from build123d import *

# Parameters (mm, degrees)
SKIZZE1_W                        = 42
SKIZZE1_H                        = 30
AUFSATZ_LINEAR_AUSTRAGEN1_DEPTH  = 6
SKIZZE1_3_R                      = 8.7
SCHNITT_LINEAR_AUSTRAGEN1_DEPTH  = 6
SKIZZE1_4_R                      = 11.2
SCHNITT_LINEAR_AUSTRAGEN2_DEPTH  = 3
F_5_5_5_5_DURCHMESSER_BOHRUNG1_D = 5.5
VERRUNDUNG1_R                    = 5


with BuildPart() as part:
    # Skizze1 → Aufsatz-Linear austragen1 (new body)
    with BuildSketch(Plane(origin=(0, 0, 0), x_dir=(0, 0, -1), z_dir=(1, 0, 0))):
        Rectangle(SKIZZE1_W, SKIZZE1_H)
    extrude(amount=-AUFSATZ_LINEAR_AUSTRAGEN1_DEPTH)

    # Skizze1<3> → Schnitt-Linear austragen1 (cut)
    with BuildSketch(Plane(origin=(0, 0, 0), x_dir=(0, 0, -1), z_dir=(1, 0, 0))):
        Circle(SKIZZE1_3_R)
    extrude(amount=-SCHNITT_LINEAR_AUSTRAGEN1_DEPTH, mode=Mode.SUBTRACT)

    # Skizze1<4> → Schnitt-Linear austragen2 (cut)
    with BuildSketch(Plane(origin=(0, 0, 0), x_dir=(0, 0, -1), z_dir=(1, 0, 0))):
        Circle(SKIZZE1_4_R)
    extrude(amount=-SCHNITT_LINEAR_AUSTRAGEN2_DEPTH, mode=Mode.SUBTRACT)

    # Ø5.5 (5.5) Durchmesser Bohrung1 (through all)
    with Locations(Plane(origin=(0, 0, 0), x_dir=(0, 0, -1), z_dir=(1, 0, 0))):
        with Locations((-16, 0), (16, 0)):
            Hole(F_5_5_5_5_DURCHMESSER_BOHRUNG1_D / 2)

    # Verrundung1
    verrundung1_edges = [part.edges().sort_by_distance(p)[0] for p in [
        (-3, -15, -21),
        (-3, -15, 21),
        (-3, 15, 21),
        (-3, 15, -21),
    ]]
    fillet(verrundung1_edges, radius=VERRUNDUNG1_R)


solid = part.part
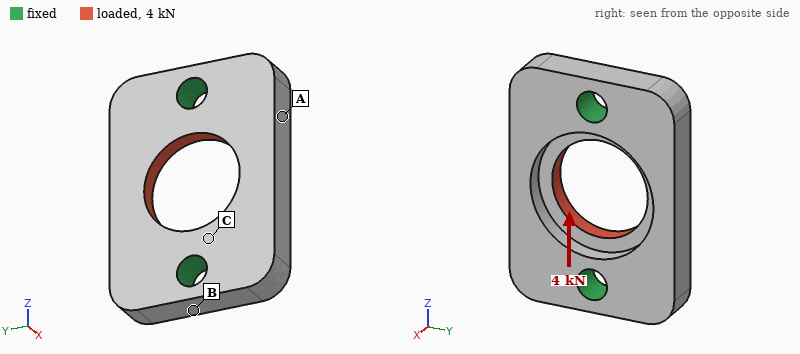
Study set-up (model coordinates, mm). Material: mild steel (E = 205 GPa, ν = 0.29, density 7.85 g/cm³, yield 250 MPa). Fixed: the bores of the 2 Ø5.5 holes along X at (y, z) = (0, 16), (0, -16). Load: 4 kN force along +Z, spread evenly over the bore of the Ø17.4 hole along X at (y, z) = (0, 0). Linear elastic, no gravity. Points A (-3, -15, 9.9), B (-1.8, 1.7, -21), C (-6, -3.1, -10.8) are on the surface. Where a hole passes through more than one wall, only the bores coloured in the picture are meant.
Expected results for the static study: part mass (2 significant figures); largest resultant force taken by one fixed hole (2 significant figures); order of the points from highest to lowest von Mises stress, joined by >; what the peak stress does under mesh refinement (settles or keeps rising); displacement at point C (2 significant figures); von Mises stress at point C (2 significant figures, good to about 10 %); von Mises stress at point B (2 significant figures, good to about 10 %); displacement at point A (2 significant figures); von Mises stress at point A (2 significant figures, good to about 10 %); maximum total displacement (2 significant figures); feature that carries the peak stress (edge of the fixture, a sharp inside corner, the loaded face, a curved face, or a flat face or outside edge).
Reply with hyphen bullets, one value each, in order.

- 41 g
- 2.0 kN
- C > B > A
- keeps rising
- 1.0 µm
- 46 MPa
- 27 MPa
- 2.3 µm
- 8.6 MPa
- 3.3 µm
- edge of the fixture
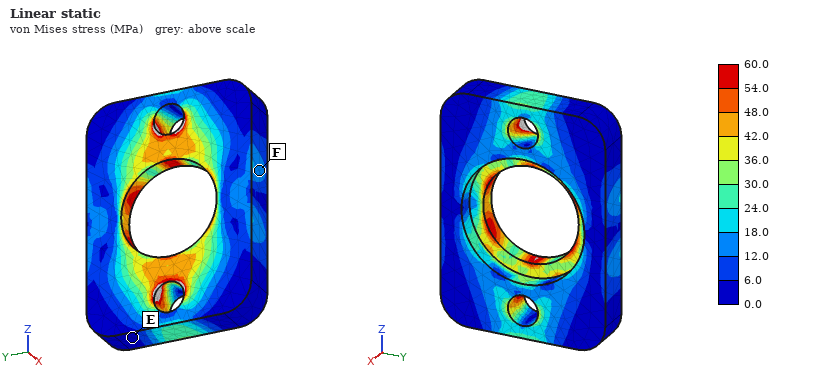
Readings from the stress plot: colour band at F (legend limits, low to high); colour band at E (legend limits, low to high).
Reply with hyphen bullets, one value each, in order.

- 12.0 to 18.0 MPa
- 0.0 to 6.0 MPa
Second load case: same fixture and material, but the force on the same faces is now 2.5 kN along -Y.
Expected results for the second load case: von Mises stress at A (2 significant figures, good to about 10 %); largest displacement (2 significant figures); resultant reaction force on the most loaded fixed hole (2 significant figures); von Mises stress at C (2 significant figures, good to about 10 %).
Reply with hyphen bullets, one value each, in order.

- 7.5 MPa
- 3.5 µm
- 1.3 kN
- 30 MPa
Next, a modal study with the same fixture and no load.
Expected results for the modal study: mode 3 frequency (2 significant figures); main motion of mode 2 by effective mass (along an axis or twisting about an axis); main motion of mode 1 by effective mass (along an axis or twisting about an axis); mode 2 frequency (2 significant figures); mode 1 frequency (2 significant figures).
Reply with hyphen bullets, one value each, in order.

- 26 kHz
- along X
- twisting about Z
- 17 kHz
- 16 kHz
